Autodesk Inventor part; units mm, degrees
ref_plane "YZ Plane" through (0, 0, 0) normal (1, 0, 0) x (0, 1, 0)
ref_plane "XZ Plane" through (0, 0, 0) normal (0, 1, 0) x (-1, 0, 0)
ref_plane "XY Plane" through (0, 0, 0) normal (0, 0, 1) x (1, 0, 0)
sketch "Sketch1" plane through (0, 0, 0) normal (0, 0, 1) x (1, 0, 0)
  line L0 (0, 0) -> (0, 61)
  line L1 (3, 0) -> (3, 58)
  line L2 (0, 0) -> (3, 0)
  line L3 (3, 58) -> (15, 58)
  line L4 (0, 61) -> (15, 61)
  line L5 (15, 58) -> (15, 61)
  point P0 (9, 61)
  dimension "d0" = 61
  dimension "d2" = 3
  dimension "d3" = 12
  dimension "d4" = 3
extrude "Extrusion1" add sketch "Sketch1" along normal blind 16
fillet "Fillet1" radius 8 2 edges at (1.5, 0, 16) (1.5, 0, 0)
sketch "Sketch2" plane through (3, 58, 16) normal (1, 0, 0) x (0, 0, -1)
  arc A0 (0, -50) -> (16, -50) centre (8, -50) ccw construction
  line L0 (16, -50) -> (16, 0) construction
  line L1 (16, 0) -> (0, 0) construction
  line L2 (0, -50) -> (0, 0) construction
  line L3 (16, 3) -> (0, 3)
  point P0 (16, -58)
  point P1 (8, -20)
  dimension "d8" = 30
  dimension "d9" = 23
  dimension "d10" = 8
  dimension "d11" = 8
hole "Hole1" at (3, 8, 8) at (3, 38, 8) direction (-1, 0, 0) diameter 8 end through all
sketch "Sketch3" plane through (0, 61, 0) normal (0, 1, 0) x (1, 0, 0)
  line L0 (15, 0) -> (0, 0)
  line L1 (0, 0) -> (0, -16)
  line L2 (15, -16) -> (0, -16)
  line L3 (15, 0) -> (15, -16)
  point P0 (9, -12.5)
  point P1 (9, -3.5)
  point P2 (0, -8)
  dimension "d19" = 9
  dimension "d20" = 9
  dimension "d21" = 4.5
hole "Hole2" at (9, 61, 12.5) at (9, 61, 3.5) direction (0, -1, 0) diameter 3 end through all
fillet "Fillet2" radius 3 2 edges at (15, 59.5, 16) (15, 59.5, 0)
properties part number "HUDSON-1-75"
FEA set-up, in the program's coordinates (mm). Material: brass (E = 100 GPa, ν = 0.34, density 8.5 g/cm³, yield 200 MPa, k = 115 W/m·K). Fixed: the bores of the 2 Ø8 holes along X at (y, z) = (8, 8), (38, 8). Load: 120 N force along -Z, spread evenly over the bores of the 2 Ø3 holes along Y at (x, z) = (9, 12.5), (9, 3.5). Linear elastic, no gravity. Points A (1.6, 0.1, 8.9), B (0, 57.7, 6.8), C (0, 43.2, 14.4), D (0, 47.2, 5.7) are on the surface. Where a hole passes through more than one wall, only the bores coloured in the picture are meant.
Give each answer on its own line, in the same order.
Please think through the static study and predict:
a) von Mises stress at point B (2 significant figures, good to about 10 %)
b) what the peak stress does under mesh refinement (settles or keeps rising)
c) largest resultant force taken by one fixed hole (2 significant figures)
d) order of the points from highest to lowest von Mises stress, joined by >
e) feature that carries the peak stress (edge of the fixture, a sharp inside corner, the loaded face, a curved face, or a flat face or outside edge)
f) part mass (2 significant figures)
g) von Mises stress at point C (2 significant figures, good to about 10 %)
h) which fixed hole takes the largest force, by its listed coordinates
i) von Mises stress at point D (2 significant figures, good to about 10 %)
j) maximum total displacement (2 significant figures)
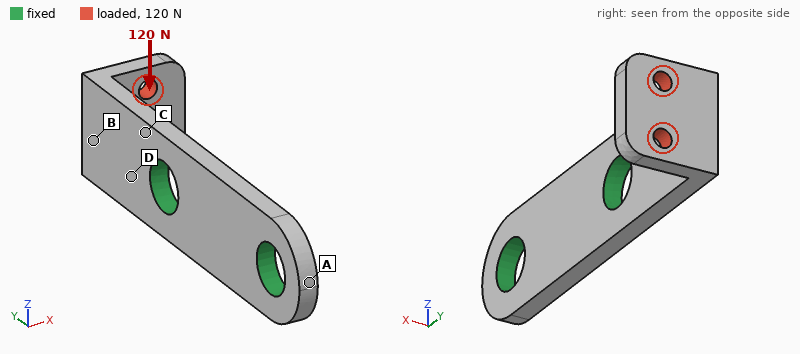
18 MPa
keeps rising
130 N
C > D > B > A
edge of the fixture
26 g
30 MPa
(38, 8)
24 MPa
45 µm
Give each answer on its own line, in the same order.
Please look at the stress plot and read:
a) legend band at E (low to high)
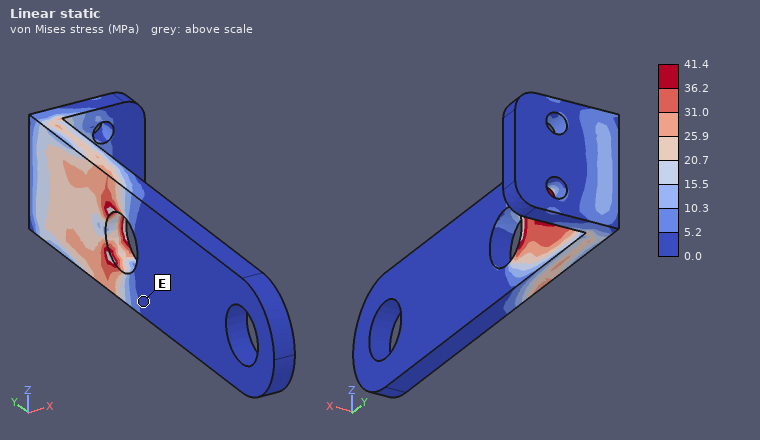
0.0 to 5.2 MPa
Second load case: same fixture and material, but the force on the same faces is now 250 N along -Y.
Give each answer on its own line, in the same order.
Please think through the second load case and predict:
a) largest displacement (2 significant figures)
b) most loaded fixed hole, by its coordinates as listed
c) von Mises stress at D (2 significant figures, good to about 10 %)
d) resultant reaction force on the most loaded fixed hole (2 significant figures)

0.17 mm
(38, 8)
67 MPa
240 N
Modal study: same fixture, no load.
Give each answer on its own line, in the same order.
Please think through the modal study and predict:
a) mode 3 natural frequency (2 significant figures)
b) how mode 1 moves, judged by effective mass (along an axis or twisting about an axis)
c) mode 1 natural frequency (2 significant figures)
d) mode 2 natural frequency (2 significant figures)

7000 Hz
along X
2200 Hz
4100 Hz
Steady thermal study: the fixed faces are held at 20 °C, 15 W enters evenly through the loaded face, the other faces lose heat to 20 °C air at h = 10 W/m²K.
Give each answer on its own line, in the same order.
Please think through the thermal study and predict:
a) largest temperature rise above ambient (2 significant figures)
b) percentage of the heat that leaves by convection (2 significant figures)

72 K
3.4 %
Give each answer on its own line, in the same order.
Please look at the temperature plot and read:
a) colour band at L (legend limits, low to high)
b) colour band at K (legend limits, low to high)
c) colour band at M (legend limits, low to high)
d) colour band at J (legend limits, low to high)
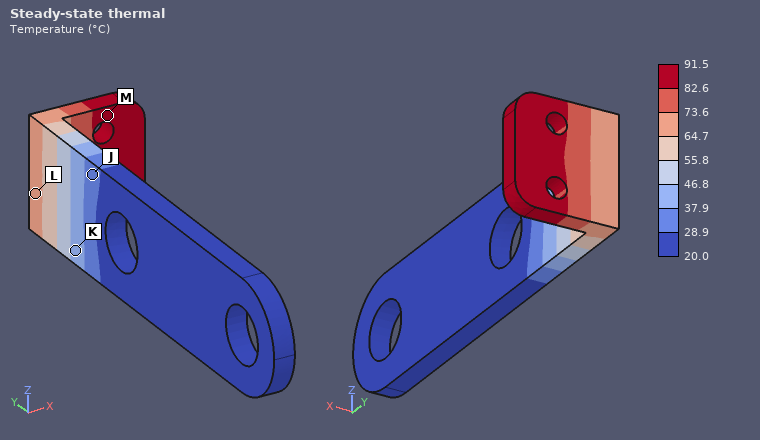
64.7 to 73.6 °C
37.9 to 46.8 °C
82.6 to 91.5 °C
28.9 to 37.9 °C
